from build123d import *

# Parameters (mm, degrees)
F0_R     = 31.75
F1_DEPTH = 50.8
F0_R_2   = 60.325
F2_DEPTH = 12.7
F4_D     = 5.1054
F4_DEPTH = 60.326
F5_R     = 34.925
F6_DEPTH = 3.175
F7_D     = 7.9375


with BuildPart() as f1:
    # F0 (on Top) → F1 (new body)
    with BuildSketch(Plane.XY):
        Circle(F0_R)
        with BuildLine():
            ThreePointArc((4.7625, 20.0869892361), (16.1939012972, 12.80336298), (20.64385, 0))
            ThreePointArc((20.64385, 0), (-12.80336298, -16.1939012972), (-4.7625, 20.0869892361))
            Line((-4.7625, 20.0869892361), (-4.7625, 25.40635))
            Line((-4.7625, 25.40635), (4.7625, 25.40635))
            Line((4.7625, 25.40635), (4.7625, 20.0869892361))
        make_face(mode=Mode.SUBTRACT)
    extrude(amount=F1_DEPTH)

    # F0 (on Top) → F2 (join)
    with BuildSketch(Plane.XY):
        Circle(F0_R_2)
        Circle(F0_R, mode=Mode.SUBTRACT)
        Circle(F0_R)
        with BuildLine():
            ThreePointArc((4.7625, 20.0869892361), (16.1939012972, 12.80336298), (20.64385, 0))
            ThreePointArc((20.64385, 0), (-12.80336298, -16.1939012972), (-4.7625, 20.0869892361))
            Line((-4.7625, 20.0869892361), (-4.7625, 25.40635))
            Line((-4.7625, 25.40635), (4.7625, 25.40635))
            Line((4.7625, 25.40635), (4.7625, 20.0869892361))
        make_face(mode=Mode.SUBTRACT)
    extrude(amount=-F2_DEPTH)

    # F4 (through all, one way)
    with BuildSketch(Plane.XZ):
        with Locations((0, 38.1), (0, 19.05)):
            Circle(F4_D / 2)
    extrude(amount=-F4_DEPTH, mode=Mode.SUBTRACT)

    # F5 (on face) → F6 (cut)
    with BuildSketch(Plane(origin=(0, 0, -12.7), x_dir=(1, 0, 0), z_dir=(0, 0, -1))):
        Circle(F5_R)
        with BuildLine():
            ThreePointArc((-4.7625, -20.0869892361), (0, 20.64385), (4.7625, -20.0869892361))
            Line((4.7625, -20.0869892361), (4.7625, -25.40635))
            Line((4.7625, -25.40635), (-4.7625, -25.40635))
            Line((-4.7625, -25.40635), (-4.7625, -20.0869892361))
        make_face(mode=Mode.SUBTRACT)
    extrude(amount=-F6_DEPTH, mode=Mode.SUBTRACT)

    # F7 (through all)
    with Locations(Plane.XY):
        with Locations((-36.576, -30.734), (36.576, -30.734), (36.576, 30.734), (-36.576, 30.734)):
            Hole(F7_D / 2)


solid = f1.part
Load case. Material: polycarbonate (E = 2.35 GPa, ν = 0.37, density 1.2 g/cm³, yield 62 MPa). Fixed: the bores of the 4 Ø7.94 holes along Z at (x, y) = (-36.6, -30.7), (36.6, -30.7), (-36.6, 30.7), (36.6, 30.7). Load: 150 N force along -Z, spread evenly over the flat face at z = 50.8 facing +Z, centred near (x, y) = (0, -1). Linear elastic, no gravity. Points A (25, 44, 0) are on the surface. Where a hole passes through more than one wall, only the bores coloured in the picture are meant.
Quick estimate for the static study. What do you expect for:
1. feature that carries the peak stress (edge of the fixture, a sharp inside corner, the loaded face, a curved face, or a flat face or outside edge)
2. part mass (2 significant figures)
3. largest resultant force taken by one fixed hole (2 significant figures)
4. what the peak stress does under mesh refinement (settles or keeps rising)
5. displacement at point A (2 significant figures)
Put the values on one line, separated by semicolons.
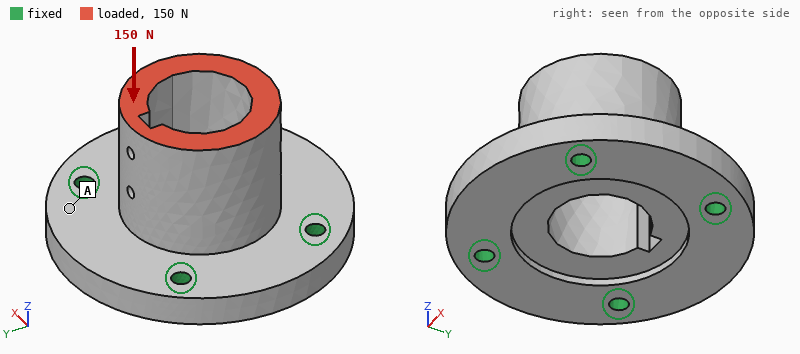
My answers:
edge of the fixture; 250 g; 42 N; keeps rising; 1.3 µm
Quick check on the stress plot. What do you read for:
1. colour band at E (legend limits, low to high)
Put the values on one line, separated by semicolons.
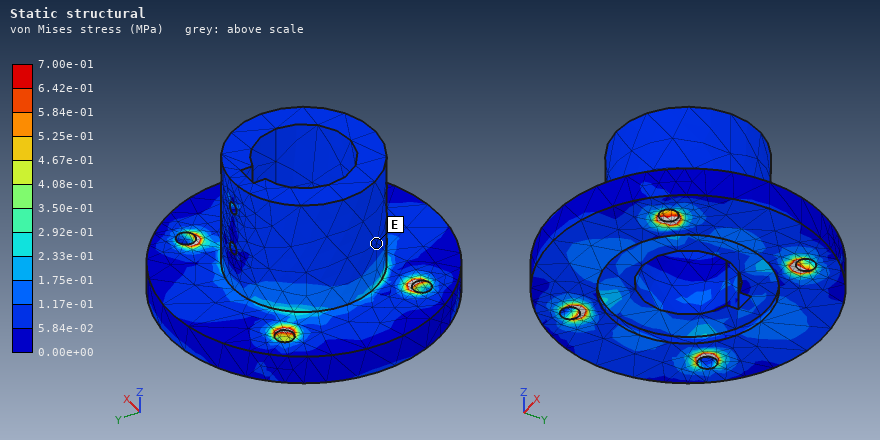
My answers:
5.84e-02 to 1.17e-01 MPa
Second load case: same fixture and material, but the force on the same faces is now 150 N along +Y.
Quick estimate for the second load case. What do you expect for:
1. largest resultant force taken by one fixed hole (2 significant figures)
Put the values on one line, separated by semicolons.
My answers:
85 N
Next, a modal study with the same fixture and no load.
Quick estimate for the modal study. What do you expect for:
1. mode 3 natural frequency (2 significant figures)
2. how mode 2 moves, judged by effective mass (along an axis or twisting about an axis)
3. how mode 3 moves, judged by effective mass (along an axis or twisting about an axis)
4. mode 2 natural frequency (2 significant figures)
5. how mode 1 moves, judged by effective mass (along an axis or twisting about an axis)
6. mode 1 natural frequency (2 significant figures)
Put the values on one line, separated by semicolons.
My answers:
2000 Hz; along X; along Z; 1600 Hz; along Y; 1400 Hz
